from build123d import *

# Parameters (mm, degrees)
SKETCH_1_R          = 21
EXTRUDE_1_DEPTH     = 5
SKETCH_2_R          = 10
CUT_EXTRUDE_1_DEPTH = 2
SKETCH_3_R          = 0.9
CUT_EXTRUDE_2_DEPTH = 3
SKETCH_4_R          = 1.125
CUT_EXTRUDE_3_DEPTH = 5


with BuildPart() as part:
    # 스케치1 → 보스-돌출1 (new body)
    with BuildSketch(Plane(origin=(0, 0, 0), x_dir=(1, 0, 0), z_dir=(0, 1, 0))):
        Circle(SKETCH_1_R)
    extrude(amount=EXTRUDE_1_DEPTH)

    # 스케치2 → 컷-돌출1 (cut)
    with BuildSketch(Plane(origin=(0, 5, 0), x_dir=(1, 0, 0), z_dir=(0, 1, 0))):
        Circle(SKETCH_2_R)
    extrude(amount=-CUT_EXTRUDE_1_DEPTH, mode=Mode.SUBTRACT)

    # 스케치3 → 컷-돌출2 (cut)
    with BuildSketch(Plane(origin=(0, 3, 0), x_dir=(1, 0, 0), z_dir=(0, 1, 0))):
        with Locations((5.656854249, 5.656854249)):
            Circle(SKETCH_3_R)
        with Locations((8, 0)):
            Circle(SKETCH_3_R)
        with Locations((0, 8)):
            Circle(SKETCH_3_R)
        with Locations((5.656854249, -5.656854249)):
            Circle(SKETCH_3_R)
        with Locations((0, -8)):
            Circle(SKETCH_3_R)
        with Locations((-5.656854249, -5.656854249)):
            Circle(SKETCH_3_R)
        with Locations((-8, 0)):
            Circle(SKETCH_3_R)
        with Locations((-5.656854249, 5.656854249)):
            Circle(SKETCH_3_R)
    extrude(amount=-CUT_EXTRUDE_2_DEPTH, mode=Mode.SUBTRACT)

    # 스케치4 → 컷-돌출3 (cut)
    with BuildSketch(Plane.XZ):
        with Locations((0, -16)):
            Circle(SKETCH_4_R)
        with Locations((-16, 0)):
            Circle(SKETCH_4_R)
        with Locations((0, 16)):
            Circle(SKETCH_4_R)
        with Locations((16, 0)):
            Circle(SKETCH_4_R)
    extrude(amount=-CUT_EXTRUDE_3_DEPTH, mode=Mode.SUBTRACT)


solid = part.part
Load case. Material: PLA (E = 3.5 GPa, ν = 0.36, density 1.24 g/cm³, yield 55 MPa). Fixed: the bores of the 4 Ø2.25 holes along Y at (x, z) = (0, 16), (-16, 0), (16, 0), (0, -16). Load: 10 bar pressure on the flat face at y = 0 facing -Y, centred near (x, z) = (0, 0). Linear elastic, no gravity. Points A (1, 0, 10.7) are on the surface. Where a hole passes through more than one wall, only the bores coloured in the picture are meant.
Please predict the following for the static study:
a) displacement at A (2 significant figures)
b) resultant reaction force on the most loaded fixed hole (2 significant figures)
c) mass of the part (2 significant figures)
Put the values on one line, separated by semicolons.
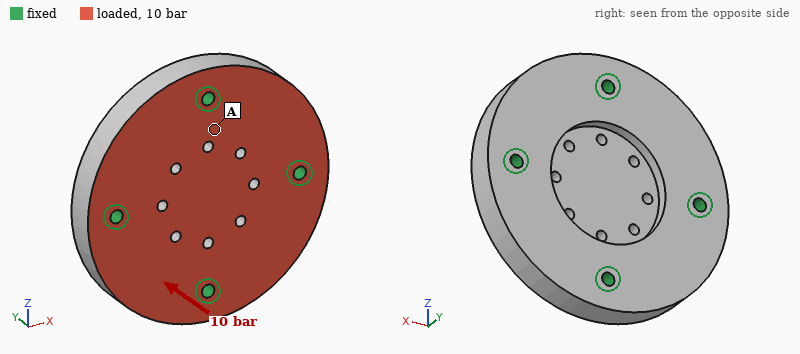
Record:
36 µm; 340 N; 7.6 g
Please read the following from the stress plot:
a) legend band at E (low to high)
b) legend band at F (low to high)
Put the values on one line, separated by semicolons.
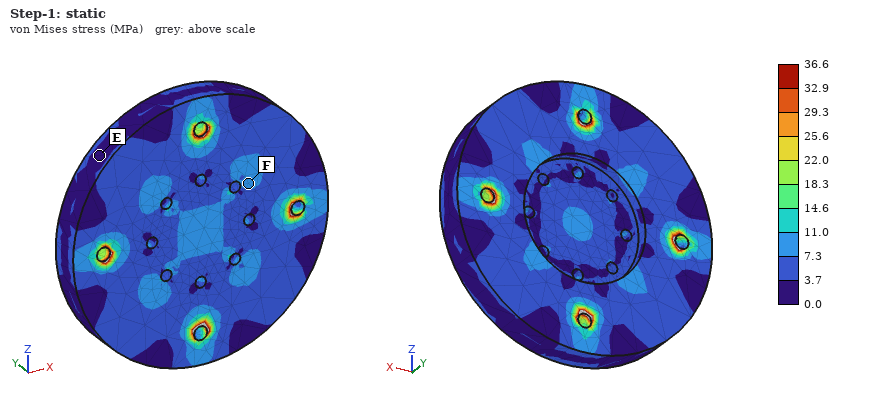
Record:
0.0 to 3.7 MPa; 7.3 to 11.0 MPa
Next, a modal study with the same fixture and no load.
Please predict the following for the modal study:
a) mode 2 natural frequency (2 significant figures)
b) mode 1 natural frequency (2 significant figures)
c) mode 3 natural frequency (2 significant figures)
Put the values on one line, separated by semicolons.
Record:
9300 Hz; 8400 Hz; 9300 Hz
